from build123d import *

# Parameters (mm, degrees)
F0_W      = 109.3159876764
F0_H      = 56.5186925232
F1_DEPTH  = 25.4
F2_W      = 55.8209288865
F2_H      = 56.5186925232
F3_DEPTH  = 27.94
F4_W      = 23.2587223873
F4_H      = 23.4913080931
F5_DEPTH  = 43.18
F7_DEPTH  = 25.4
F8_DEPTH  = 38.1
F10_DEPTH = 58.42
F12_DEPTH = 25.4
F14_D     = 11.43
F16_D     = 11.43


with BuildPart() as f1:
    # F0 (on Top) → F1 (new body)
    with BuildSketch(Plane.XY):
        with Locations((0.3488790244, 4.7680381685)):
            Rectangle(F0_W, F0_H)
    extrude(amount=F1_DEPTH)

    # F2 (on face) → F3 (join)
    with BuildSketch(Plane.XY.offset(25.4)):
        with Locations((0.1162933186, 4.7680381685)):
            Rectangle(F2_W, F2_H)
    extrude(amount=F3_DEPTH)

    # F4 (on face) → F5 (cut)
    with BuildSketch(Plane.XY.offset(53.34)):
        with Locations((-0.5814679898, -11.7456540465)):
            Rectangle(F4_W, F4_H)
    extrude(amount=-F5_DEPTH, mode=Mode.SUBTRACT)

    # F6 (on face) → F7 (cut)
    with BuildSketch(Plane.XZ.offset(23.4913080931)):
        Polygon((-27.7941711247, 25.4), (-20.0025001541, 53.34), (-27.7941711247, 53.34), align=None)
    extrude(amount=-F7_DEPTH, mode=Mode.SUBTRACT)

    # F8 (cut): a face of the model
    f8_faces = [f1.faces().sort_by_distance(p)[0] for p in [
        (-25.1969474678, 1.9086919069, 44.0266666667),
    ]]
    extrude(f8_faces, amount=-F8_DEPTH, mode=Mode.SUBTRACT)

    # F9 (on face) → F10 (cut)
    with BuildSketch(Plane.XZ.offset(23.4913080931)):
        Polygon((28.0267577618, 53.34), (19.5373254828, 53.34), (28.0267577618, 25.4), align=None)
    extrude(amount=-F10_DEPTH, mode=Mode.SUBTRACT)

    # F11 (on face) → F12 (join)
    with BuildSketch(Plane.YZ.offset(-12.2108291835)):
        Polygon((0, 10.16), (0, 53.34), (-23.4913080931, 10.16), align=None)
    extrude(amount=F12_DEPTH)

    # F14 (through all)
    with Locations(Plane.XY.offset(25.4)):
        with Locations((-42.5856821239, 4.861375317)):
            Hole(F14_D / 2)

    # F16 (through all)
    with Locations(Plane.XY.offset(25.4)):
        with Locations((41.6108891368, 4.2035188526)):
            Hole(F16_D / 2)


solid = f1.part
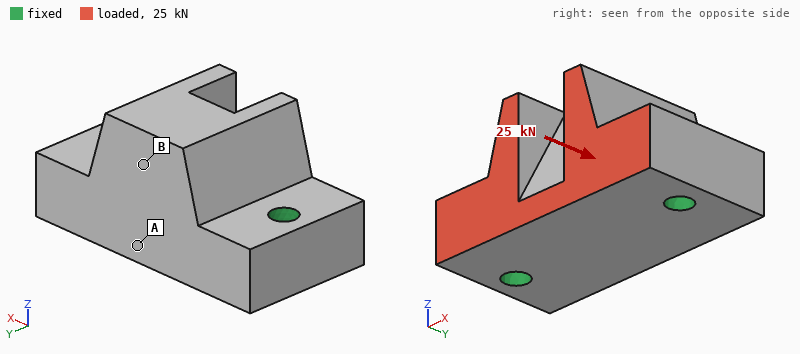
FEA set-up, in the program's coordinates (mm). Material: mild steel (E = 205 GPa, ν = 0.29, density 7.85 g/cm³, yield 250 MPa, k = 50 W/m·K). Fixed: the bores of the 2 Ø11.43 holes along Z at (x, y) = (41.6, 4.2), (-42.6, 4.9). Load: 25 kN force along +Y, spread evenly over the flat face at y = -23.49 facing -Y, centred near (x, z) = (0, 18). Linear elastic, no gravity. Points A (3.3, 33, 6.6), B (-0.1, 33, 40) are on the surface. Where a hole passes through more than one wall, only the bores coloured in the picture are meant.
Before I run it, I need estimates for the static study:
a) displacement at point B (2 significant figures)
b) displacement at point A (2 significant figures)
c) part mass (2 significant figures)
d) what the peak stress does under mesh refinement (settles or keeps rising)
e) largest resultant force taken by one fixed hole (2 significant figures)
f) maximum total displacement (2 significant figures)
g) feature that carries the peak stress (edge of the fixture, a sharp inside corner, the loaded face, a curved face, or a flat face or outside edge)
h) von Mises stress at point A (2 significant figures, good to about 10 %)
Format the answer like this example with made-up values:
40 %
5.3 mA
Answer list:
6.0 µm
3.1 µm
1.7 kg
keeps rising
13 kN
8.4 µm
edge of the fixture
11 MPa
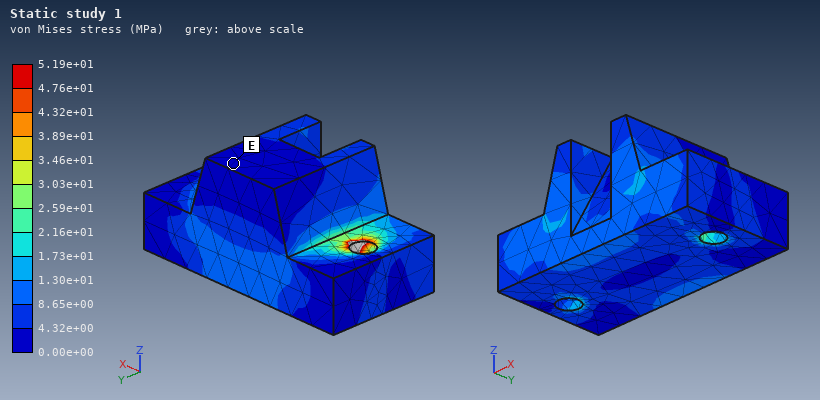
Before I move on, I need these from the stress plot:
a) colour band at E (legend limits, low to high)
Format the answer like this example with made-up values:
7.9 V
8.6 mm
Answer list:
0.00e+00 to 4.32e+00 MPa
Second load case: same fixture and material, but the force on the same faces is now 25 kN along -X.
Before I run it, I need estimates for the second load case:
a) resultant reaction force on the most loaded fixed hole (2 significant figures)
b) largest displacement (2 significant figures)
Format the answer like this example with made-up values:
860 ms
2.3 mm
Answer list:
15 kN
13 µm
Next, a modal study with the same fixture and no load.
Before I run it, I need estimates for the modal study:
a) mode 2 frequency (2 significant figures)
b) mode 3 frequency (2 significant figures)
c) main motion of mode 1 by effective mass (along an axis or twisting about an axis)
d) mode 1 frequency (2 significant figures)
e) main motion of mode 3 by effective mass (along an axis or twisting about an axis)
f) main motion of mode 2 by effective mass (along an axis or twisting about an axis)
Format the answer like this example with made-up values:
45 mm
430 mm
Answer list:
10 kHz
12 kHz
along Y
6600 Hz
along Y
along Z
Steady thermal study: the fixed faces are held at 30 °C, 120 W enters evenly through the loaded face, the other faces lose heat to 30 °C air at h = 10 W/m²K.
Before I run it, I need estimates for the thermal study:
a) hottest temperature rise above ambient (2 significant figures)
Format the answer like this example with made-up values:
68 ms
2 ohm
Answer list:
33 K
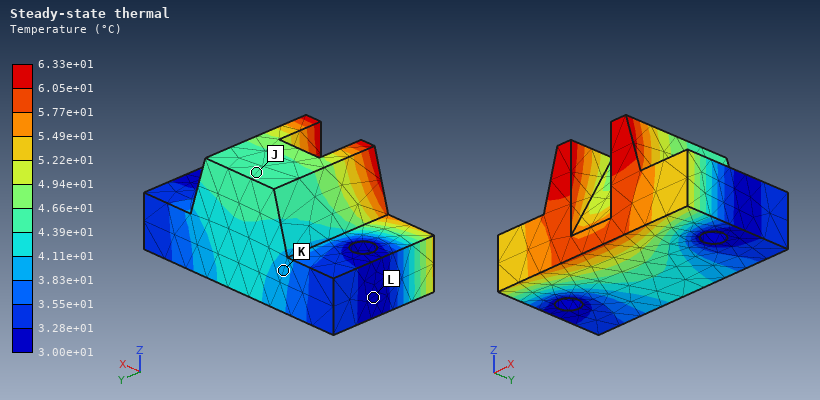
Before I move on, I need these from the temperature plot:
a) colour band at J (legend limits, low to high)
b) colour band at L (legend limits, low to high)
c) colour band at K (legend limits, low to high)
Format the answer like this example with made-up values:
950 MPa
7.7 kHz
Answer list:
4.39e+01 to 4.66e+01 °C
3.00e+01 to 3.28e+01 °C
3.83e+01 to 4.11e+01 °C
